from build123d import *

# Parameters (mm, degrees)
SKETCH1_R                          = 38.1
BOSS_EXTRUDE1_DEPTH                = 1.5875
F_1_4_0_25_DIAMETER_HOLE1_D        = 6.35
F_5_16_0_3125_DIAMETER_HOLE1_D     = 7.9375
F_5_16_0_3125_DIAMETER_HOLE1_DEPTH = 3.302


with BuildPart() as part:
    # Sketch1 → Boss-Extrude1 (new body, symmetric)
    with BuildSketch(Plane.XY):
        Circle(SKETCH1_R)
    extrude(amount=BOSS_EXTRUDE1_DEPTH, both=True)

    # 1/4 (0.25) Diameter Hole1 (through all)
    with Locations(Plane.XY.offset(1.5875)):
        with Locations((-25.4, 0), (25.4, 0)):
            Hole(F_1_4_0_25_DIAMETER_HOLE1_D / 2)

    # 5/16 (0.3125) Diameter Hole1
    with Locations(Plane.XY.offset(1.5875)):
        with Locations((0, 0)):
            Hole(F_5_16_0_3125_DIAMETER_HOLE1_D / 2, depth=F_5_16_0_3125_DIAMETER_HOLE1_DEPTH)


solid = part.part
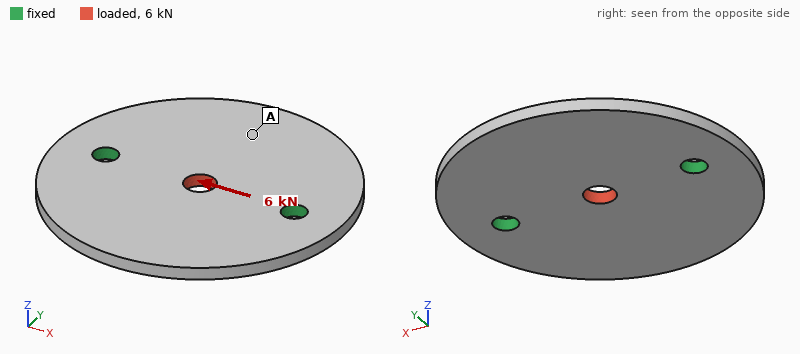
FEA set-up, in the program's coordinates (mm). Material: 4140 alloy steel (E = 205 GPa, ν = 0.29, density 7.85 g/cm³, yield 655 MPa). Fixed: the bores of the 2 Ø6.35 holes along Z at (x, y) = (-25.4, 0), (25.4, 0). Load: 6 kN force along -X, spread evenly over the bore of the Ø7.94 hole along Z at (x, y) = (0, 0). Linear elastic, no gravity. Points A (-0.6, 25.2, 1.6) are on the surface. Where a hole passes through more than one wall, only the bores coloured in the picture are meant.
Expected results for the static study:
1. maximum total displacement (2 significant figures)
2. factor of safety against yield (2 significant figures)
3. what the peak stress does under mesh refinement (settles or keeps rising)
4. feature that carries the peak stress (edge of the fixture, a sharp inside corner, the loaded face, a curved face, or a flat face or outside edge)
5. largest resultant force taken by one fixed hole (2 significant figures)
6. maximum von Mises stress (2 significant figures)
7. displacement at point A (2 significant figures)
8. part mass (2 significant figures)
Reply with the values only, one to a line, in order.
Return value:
6.1 µm
5.0
settles
the loaded face
3.0 kN
130 MPa
2.4 µm
110 g
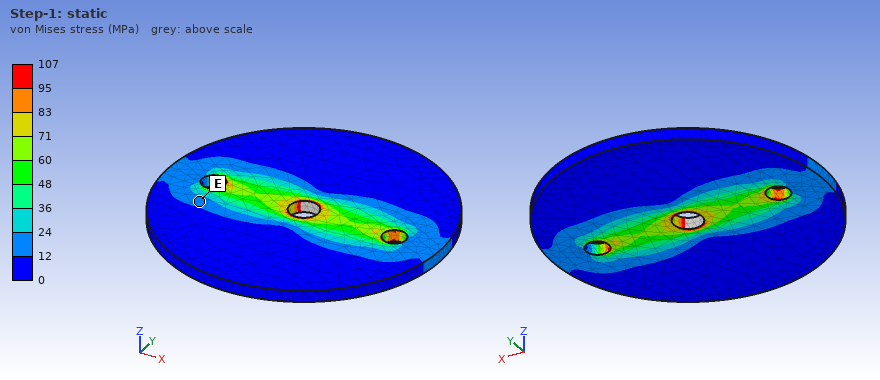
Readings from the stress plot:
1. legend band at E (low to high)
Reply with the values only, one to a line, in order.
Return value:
12 to 24 MPa
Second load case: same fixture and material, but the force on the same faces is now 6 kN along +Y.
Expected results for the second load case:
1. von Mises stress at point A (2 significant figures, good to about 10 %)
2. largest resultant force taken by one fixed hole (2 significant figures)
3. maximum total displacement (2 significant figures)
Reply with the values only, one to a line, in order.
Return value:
20 MPa
3.0 kN
8.5 µm
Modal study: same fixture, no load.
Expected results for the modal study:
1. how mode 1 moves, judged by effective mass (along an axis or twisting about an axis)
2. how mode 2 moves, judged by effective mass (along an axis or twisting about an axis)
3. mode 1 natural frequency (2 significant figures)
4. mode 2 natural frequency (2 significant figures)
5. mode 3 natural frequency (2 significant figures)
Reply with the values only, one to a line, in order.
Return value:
twisting about X
along Z
2000 Hz
2300 Hz
5000 Hz
